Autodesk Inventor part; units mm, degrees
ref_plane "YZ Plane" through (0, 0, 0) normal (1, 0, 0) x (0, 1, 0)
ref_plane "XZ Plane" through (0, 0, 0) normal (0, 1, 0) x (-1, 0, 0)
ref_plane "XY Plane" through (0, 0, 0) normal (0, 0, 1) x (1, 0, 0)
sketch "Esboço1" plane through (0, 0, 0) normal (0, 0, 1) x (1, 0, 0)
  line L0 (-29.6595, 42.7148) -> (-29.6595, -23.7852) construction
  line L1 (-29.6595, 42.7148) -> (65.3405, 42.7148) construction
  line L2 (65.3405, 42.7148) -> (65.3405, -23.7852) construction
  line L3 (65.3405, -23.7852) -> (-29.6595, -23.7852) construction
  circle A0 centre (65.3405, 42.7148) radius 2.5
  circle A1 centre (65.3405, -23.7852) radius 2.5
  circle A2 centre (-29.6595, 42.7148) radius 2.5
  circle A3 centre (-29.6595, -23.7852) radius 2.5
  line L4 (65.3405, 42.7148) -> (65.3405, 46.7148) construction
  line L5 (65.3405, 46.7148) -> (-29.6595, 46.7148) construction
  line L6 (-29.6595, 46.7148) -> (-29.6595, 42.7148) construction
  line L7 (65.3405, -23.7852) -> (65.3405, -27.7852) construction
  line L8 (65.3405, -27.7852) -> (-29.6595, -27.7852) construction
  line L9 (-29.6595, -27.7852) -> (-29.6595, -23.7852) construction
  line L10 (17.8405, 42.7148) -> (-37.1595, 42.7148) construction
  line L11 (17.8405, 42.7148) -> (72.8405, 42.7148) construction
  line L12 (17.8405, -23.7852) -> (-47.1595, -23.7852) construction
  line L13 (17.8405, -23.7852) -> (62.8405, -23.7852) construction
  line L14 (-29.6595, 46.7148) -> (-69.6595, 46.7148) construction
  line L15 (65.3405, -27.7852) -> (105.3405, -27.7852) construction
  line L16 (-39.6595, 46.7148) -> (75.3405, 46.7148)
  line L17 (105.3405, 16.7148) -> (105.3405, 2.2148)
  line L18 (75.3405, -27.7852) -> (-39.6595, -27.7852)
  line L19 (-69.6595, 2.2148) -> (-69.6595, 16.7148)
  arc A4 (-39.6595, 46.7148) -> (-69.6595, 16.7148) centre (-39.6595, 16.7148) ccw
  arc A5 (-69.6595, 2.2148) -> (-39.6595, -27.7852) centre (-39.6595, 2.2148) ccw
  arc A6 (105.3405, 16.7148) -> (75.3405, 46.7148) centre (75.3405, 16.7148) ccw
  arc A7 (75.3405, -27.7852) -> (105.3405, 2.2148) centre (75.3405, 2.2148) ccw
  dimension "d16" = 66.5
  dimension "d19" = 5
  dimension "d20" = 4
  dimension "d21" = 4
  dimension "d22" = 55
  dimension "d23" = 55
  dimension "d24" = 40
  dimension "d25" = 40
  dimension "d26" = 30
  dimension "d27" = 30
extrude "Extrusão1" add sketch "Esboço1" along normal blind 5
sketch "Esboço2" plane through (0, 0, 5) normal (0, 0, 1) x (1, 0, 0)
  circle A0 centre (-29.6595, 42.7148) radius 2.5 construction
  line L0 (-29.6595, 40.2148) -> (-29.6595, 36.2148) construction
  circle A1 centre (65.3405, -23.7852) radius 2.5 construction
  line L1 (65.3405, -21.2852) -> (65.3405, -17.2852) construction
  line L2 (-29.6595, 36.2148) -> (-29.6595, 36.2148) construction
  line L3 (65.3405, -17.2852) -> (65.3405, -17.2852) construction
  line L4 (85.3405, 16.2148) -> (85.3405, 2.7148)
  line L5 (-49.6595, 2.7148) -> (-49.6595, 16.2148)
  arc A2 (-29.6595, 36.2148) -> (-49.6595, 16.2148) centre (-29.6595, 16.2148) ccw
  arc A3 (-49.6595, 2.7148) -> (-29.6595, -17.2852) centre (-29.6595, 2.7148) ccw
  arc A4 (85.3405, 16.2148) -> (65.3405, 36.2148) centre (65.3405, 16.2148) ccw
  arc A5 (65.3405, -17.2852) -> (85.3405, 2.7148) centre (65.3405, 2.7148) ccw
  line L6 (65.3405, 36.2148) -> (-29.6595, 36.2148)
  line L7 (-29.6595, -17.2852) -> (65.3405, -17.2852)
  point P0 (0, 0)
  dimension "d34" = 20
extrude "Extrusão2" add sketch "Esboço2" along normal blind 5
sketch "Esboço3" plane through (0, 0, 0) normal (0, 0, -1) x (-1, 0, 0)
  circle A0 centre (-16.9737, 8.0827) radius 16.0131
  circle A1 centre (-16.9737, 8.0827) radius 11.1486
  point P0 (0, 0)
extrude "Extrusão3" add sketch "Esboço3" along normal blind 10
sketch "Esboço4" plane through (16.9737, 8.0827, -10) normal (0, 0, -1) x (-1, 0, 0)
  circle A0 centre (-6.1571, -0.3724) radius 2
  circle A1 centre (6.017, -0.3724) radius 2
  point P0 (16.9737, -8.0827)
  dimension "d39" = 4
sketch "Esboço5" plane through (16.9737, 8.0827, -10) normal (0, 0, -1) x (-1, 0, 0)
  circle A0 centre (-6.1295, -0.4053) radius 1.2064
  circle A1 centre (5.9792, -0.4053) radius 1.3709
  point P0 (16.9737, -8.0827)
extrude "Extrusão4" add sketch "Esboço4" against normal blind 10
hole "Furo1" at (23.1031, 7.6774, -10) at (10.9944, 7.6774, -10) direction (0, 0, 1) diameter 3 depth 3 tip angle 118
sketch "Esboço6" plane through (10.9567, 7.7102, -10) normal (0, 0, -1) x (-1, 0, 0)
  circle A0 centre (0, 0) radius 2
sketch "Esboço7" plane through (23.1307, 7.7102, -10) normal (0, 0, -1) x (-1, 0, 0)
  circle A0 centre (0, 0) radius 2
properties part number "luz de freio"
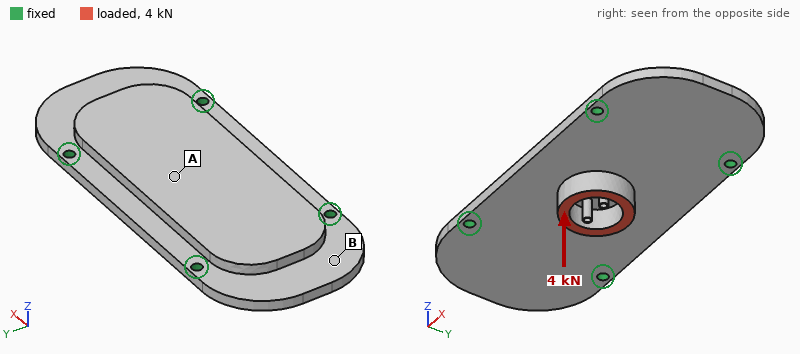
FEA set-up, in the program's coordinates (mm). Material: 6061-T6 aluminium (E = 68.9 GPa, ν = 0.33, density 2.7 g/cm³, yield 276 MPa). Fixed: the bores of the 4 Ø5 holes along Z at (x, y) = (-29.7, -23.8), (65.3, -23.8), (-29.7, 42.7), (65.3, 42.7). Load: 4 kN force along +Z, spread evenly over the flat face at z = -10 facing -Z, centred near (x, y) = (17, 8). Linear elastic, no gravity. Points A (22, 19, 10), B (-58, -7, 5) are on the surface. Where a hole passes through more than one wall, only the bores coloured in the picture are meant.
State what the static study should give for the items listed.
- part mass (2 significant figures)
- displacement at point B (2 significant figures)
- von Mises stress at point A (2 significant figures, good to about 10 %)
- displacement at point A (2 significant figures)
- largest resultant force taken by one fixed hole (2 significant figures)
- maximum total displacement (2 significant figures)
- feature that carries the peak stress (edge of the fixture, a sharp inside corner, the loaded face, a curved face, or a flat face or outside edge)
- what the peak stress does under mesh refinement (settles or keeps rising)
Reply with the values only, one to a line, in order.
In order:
270 g
0.045 mm
40 MPa
0.10 mm
1.7 kN
0.11 mm
edge of the fixture
keeps rising
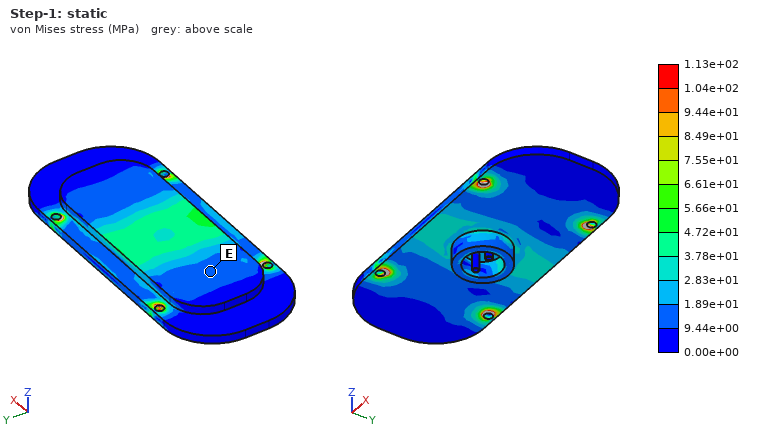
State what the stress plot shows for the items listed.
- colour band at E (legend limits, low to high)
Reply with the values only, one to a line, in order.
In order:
9.44e+00 to 1.89e+01 MPa
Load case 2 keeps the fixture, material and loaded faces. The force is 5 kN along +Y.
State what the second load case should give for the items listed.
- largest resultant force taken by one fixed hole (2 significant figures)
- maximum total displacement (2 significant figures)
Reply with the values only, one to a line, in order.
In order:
1.6 kN
79 µm
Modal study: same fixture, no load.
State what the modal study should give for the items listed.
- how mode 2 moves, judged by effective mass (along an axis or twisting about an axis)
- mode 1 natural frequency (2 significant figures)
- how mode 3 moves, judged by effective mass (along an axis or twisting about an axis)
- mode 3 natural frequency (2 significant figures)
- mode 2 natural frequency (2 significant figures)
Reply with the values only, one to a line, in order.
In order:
twisting about Y
2800 Hz
along Z
3900 Hz
3600 Hz
